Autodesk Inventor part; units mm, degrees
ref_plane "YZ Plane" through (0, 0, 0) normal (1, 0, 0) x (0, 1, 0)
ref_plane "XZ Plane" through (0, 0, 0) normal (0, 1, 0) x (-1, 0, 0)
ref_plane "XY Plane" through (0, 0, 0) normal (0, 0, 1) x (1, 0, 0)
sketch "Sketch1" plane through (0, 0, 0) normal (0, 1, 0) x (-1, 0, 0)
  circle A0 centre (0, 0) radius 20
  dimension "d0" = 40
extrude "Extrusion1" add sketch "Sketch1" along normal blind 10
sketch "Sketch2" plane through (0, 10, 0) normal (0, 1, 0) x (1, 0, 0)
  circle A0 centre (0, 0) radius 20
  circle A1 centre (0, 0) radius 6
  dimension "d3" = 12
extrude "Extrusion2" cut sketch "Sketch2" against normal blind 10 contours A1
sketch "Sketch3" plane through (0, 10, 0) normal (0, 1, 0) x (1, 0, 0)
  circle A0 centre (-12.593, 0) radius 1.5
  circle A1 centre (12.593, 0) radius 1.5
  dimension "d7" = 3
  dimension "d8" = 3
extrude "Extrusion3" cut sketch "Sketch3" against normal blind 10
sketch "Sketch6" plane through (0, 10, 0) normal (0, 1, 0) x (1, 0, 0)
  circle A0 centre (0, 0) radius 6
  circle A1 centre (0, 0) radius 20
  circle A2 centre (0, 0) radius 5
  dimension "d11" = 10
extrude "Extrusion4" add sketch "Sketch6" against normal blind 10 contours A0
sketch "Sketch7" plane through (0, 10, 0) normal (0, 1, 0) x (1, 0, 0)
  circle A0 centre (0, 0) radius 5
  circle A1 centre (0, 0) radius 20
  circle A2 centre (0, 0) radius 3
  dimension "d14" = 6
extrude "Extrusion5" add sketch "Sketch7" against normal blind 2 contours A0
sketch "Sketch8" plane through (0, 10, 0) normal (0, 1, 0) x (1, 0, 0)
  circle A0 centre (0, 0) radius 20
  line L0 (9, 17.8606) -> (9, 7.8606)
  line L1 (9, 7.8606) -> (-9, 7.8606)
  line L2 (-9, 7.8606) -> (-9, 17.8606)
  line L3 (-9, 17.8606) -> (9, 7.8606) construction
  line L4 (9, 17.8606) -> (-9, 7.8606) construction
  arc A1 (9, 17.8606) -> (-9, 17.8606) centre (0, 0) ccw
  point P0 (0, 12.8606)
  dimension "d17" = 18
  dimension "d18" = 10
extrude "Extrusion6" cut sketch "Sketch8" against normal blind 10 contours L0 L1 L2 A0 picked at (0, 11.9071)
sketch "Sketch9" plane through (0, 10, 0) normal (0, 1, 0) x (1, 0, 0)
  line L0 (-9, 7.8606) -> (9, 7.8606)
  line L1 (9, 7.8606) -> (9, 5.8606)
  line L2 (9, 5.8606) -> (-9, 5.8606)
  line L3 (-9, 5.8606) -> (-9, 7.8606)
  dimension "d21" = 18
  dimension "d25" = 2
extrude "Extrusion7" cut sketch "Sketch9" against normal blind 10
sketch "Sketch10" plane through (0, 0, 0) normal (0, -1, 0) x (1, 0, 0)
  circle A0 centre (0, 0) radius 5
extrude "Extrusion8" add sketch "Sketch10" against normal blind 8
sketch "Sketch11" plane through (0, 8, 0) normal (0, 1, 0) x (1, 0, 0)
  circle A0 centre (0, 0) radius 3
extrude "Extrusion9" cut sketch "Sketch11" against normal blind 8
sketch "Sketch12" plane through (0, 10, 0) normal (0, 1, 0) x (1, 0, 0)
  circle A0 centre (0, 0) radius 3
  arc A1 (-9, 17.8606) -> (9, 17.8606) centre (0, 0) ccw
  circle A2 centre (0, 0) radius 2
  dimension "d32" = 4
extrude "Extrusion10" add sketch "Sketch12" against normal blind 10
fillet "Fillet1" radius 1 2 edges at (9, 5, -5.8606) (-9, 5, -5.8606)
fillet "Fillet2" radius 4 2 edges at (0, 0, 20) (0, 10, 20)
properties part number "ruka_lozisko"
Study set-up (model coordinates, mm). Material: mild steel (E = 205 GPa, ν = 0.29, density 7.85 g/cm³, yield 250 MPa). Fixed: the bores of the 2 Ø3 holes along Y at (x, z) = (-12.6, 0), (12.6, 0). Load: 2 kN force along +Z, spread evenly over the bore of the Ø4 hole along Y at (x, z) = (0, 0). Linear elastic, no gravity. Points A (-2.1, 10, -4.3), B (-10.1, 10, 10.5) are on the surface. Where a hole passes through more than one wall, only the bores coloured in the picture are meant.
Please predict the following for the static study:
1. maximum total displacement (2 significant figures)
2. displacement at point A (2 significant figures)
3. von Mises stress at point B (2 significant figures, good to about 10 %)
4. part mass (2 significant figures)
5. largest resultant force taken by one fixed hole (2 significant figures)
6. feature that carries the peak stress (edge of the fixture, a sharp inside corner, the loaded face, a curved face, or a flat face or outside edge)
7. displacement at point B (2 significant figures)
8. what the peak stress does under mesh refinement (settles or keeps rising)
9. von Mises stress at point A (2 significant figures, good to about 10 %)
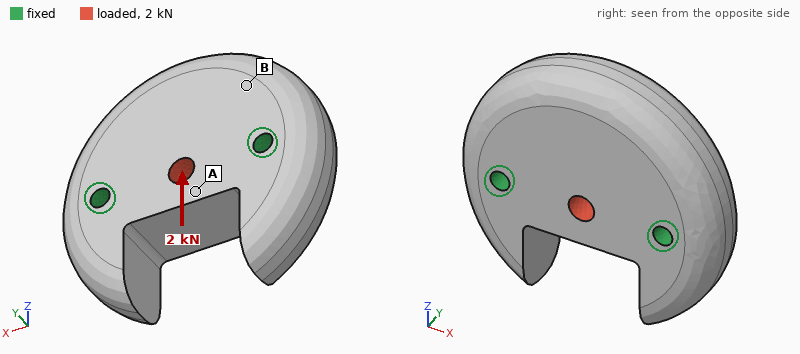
1.5 µm
1.3 µm
6.1 MPa
72 g
1.0 kN
edge of the fixture
0.44 µm
keeps rising
15 MPa
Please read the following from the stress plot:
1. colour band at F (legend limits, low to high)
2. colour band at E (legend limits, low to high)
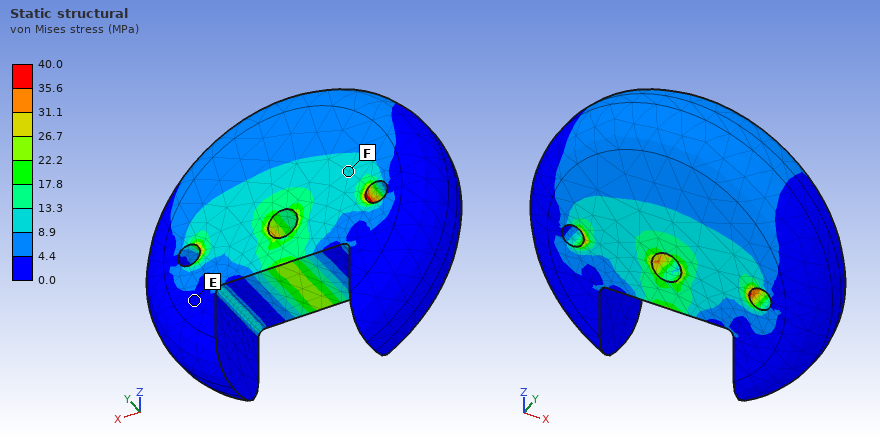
8.9 to 13.3 MPa
0.0 to 4.4 MPa
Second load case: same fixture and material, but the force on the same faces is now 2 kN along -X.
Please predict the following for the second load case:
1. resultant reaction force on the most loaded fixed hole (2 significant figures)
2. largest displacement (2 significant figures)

1.0 kN
0.68 µm
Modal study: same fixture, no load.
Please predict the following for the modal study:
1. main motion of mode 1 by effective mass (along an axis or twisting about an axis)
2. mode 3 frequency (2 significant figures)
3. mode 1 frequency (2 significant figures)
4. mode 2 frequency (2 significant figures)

along Y
33 kHz
18 kHz
33 kHz
